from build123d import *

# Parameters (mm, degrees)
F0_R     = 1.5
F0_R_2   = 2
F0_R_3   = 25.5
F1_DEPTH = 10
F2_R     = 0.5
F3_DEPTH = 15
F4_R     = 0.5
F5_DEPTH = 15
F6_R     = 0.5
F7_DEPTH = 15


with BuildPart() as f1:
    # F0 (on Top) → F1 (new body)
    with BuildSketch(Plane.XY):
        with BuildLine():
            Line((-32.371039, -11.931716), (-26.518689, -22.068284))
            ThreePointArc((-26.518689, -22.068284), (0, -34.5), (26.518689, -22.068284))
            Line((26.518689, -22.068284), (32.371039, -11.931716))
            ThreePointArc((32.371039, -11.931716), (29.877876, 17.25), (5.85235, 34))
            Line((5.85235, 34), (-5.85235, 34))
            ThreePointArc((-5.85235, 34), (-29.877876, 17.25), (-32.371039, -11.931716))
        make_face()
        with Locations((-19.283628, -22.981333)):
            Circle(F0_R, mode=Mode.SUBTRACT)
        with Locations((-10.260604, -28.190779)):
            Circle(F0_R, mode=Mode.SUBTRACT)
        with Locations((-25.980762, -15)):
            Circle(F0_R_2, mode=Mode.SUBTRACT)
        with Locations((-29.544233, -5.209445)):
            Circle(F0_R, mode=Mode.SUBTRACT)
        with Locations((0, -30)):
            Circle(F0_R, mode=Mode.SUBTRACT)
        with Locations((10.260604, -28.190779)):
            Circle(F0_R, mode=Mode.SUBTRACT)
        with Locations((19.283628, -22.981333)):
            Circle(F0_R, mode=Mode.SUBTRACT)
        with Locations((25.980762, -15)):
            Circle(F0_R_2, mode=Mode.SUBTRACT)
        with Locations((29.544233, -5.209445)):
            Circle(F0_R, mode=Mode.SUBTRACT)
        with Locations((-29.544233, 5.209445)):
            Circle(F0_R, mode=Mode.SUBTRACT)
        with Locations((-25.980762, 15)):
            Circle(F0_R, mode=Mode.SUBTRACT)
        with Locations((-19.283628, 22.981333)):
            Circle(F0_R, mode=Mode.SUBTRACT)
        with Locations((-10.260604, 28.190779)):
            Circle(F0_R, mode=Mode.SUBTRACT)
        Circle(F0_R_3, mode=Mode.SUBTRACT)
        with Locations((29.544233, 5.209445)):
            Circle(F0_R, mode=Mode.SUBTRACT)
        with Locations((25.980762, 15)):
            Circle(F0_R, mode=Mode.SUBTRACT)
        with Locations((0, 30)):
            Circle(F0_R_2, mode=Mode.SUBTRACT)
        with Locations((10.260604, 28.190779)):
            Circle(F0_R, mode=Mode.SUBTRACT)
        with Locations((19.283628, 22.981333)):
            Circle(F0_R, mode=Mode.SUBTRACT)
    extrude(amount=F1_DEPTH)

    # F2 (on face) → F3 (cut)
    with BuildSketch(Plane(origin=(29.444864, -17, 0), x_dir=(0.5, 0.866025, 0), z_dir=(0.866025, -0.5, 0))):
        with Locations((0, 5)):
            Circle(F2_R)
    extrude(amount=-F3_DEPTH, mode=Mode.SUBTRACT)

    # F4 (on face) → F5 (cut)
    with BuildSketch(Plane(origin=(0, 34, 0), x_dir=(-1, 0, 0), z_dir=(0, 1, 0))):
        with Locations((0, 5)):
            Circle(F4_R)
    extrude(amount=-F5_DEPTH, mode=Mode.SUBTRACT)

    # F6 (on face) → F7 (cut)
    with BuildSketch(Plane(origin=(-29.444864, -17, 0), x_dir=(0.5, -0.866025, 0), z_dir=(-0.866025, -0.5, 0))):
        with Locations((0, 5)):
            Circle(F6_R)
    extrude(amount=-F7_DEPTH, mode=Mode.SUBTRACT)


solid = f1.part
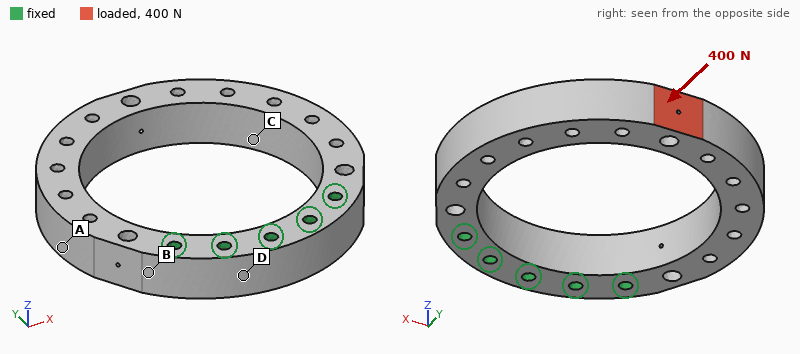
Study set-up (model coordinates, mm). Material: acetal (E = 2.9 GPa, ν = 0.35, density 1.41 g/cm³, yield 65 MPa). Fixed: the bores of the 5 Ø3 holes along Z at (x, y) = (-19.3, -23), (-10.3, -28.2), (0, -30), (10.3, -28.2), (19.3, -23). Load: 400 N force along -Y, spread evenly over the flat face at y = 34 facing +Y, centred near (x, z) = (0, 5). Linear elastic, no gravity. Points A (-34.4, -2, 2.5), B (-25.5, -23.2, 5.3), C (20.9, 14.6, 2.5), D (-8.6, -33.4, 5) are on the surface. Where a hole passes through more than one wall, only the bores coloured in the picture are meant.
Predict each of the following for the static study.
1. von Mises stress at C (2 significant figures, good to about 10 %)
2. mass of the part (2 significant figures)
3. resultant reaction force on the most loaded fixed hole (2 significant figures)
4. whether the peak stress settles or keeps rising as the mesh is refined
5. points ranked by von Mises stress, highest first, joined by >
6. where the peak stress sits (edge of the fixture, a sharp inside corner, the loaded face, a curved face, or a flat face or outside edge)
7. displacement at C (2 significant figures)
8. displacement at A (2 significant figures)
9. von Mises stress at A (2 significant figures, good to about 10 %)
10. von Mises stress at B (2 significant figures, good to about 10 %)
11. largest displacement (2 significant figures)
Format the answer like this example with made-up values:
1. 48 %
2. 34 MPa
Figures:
1. 12 MPa
2. 22 g
3. 290 N
4. keeps rising
5. C > B > A > D
6. a sharp inside corner
7. 0.29 mm
8. 0.26 mm
9. 6.5 MPa
10. 9.6 MPa
11. 0.51 mm
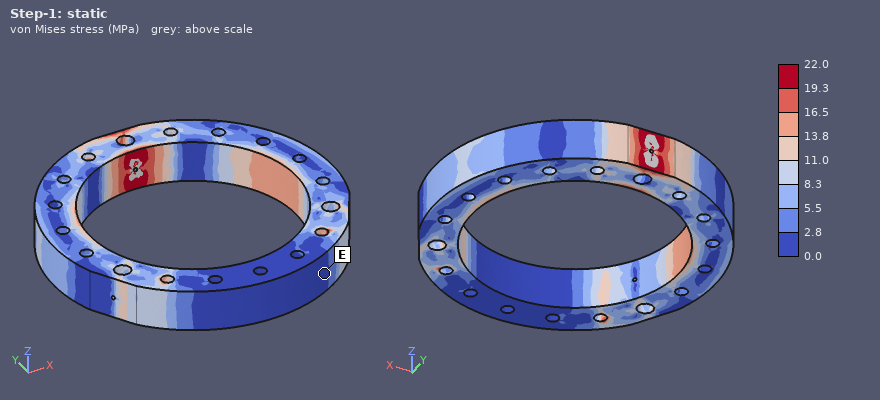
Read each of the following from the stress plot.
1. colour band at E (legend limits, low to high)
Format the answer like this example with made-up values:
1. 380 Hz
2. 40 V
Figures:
1. 0.0 to 2.8 MPa
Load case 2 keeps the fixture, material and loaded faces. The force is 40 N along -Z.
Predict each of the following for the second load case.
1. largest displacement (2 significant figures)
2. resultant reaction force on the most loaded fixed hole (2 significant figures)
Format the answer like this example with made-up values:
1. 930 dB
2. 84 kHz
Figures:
1. 1.1 mm
2. 27 N
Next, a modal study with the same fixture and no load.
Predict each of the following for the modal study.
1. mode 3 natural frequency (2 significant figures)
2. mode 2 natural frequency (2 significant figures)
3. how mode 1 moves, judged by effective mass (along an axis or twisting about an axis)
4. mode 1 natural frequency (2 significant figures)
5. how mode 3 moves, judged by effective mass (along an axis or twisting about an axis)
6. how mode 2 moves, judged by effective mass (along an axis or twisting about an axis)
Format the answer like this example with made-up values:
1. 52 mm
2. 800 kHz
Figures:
1. 1100 Hz
2. 720 Hz
3. along Z
4. 440 Hz
5. twisting about Y
6. along X
